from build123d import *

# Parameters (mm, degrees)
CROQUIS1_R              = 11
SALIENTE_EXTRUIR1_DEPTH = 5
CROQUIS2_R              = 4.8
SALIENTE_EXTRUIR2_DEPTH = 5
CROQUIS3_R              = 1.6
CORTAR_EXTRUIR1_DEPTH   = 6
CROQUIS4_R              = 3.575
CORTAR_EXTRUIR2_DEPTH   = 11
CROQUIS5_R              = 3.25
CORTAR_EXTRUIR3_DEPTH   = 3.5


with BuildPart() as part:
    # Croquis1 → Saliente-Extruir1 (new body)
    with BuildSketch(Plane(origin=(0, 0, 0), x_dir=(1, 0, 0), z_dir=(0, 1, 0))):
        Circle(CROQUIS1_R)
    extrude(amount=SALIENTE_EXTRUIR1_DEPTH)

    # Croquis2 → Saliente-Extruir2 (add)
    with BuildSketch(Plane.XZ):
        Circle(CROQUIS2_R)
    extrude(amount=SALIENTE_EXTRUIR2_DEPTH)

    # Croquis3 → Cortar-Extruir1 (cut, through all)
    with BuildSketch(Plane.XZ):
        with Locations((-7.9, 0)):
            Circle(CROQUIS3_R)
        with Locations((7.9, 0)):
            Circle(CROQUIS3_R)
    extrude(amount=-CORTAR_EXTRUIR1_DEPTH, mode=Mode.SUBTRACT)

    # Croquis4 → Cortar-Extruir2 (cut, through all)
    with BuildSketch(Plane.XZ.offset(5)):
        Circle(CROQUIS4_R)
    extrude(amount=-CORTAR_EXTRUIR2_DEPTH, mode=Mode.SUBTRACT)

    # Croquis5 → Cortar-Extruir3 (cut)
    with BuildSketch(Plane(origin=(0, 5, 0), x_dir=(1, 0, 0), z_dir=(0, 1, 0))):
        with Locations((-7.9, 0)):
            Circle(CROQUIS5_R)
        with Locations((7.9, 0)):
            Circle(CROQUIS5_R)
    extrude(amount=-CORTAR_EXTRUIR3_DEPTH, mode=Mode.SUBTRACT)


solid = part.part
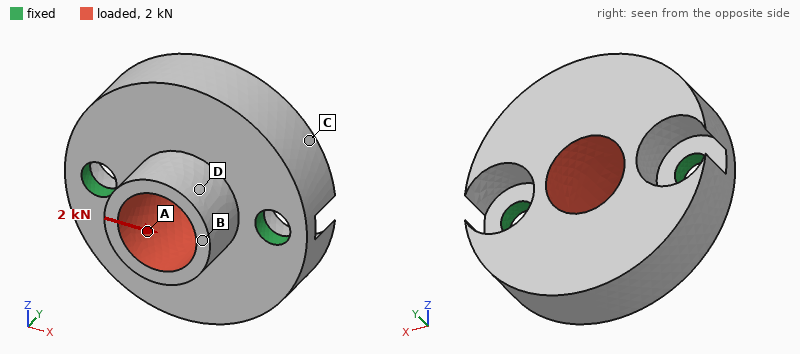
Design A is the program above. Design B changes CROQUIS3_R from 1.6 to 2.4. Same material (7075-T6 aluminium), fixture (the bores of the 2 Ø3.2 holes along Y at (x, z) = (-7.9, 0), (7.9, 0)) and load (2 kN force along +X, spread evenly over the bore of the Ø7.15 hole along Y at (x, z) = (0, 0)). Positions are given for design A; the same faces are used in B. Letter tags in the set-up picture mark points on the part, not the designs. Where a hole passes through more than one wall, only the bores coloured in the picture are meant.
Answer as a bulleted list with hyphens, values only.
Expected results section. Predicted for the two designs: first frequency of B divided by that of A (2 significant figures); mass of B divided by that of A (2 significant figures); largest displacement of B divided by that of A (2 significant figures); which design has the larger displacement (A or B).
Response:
- 1.4
- 0.98
- 0.85
- A
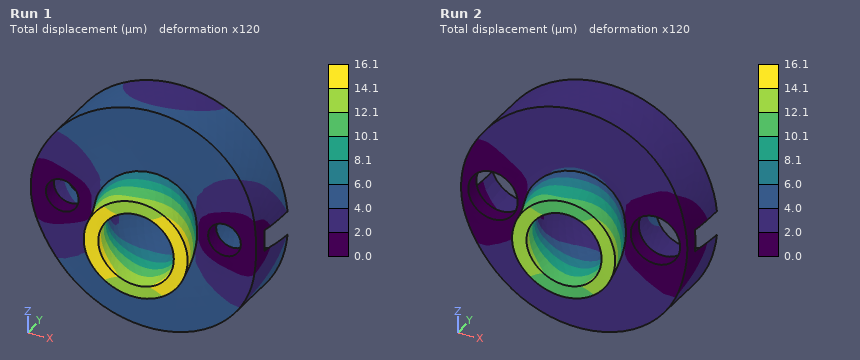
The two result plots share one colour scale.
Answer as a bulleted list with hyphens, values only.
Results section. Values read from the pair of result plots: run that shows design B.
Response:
- Run 2
